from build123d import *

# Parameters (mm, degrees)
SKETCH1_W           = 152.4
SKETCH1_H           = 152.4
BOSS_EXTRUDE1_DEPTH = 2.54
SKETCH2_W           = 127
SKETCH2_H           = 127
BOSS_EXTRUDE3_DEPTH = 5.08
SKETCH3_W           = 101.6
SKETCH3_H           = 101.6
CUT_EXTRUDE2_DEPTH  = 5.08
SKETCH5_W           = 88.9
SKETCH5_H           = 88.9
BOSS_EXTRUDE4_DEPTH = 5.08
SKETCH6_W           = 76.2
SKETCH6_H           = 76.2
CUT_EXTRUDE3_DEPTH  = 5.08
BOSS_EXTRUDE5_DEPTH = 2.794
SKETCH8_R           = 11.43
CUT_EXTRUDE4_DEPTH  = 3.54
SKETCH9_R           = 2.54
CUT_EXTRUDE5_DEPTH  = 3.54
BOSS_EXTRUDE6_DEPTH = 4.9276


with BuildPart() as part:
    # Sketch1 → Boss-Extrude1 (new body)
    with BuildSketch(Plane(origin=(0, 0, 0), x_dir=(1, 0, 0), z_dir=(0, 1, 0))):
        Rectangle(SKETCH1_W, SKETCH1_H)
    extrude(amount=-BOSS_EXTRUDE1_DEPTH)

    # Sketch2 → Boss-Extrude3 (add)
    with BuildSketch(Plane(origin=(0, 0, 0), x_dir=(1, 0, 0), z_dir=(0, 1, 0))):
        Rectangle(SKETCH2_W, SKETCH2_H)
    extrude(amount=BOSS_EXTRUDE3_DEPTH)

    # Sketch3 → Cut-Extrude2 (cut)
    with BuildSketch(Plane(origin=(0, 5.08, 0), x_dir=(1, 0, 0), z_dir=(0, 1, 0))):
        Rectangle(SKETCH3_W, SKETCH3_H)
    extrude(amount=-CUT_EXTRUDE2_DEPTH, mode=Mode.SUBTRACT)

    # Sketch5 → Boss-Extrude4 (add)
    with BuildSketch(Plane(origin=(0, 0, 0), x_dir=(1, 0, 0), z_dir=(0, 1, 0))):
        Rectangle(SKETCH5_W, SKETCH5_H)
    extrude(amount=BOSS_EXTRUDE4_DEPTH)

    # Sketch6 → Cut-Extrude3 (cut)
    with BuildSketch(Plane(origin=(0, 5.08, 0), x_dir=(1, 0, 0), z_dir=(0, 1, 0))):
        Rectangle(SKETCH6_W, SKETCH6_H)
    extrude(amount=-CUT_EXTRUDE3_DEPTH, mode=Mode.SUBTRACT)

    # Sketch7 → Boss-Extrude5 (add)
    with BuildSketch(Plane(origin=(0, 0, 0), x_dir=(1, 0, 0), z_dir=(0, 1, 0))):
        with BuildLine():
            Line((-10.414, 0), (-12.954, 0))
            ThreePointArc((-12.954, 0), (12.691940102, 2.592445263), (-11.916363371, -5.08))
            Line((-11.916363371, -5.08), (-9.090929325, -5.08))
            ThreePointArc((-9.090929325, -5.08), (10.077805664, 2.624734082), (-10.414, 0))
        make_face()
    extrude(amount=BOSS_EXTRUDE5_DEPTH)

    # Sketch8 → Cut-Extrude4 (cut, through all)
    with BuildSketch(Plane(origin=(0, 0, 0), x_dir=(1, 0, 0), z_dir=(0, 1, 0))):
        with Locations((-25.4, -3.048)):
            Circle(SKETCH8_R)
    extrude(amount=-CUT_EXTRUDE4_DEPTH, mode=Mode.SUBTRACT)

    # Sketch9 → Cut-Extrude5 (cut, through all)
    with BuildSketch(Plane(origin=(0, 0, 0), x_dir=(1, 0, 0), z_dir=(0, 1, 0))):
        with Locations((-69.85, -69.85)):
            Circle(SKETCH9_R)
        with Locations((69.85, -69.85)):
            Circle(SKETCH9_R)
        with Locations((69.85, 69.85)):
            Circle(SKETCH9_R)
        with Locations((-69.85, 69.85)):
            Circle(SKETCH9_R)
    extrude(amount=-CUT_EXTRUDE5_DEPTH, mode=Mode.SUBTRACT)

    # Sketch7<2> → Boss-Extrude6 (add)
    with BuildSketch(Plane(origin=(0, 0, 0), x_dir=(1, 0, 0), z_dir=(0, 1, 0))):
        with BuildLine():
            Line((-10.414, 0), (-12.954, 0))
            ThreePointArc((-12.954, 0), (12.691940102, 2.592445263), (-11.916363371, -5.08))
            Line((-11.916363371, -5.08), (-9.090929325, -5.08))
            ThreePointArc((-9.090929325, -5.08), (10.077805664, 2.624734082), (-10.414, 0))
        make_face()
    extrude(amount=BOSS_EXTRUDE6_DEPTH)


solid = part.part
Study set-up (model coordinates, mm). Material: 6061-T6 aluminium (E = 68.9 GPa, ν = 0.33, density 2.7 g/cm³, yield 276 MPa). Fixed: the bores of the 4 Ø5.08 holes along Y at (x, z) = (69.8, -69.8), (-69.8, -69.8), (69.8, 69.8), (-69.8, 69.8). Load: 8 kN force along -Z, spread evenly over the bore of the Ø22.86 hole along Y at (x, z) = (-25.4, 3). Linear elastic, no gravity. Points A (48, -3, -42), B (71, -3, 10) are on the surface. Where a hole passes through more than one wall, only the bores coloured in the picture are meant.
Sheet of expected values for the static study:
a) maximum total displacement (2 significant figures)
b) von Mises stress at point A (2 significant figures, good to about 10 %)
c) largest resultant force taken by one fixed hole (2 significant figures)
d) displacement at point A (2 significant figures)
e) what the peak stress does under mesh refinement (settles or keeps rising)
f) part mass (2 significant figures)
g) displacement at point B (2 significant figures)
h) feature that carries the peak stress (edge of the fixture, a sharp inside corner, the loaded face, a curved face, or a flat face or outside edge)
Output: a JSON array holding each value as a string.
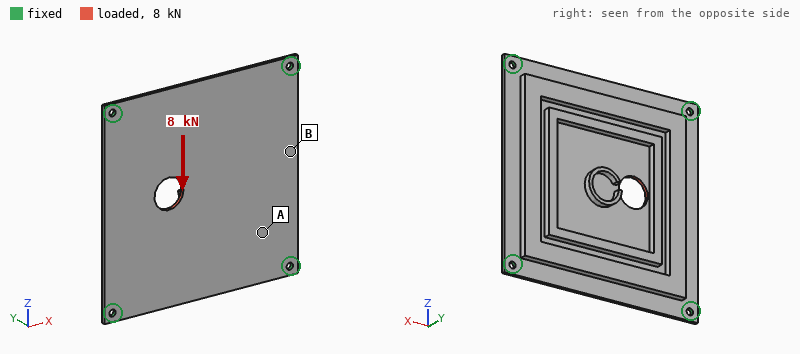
["52 µm", "18 MPa", "2.7 kN", "23 µm", "keeps rising", "270 g", "13 µm", "edge of the fixture"]
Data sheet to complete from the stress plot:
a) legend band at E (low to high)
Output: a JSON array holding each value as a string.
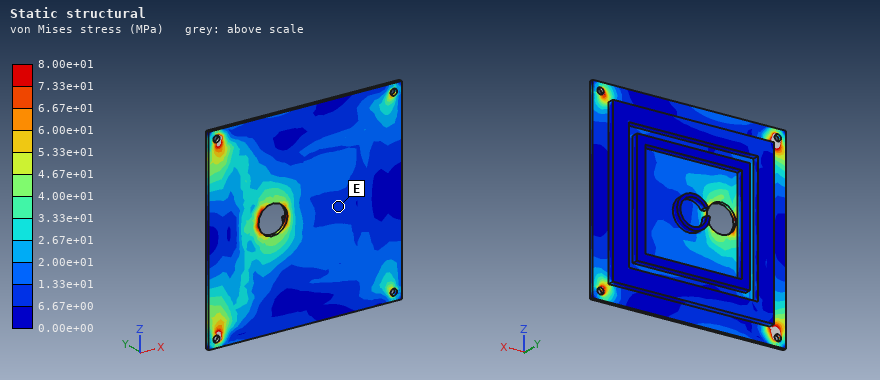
["6.67e+00 to 1.33e+01 MPa"]
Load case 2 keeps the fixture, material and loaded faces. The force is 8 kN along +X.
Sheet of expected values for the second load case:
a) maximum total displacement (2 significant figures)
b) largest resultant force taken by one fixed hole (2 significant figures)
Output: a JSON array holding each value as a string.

["75 µm", "2.4 kN"]
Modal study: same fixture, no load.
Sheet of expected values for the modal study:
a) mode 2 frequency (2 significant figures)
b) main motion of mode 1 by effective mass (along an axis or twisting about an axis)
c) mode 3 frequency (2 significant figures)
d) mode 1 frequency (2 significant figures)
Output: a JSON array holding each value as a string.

["1300 Hz", "along Y", "1300 Hz", "760 Hz"]
